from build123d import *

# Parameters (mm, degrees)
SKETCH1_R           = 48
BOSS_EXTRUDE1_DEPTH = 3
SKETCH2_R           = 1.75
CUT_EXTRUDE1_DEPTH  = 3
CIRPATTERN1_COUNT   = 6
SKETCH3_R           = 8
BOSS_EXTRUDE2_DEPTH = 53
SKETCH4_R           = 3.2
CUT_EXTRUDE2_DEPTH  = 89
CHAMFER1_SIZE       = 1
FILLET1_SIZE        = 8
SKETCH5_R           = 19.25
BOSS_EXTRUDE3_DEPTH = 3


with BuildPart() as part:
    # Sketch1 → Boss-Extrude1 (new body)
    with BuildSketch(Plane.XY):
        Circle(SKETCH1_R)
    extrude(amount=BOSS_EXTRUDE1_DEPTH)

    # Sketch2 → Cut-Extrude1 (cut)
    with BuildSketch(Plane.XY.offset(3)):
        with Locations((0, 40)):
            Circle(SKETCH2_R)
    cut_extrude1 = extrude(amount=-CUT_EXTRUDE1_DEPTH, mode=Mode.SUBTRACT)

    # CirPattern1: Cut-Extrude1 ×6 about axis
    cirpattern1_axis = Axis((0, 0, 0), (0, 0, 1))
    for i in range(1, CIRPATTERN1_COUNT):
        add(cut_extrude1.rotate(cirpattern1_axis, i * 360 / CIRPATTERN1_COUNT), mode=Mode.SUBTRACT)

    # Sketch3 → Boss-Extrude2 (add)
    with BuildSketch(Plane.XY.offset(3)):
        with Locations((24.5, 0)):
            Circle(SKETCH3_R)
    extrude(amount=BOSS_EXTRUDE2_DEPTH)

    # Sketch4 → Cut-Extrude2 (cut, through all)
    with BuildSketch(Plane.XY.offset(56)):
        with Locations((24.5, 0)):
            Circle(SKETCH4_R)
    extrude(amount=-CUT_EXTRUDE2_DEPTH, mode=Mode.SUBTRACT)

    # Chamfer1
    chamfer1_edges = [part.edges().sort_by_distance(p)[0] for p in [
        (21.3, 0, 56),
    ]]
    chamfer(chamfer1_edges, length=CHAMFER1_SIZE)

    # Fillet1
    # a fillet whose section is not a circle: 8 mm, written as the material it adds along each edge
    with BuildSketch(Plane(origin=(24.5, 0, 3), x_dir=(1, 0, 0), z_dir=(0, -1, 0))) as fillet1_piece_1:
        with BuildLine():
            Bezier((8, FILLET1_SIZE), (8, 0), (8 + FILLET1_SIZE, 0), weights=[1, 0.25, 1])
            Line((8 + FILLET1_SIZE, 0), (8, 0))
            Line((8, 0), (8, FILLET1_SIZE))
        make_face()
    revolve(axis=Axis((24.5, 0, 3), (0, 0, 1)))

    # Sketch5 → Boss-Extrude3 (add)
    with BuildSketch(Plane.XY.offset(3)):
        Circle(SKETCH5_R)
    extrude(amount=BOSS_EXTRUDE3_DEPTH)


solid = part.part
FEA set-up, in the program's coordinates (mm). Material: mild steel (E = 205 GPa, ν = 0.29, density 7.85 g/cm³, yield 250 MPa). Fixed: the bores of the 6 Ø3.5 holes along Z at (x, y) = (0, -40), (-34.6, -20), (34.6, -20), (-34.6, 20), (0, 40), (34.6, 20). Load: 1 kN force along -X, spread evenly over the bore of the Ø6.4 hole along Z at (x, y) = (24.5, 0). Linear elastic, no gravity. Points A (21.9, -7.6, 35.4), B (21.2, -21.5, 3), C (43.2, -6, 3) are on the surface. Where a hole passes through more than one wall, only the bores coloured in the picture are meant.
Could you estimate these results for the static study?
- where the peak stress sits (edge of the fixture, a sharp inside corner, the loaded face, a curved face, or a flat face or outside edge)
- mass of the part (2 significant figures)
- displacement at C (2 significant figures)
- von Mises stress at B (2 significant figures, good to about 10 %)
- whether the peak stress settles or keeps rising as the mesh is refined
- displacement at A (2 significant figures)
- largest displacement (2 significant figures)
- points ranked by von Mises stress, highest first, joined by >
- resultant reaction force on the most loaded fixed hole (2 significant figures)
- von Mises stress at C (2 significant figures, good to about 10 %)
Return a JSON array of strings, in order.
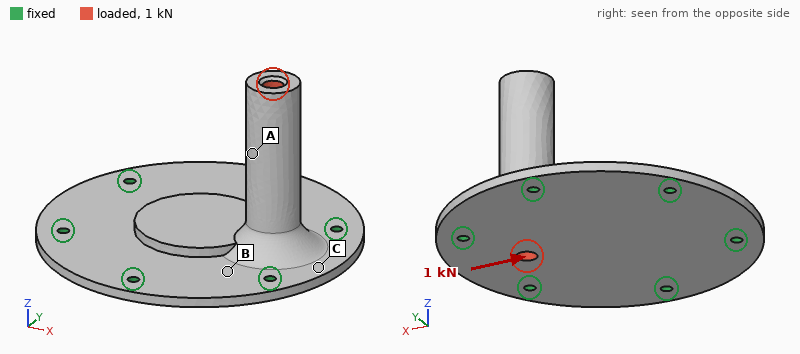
["edge of the fixture", "270 g", "14 µm", "16 MPa", "keeps rising", "48 µm", "83 µm", "C > B > A", "380 N", "25 MPa"]
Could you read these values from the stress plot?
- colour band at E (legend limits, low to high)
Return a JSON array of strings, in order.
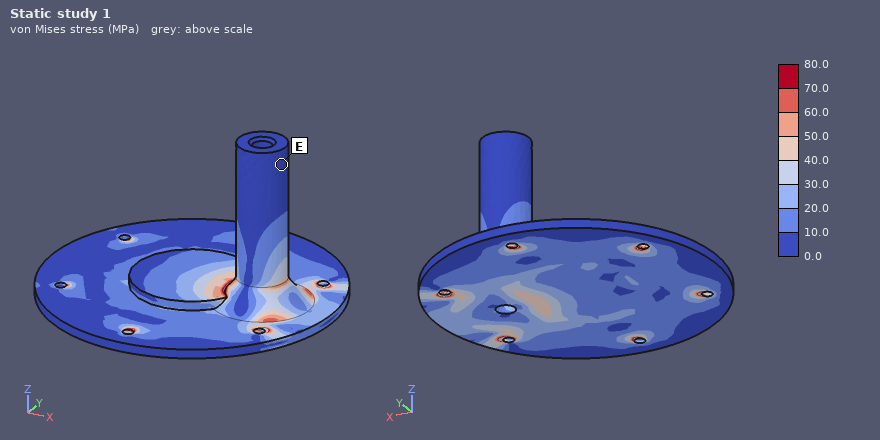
["0.0 to 10.0 MPa"]
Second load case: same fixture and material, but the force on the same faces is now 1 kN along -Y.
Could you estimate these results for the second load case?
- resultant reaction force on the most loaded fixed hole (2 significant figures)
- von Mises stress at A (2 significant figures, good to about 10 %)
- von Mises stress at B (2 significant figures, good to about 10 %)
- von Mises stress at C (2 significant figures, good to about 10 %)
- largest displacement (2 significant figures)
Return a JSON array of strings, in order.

["700 N", "8.5 MPa", "16 MPa", "15 MPa", "54 µm"]
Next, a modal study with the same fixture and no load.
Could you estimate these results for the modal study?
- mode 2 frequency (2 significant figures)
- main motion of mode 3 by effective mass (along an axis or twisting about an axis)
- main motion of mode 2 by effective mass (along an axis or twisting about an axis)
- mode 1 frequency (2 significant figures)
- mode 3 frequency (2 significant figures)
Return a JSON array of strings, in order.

["3000 Hz", "along Z", "along Y", "2300 Hz", "4900 Hz"]
